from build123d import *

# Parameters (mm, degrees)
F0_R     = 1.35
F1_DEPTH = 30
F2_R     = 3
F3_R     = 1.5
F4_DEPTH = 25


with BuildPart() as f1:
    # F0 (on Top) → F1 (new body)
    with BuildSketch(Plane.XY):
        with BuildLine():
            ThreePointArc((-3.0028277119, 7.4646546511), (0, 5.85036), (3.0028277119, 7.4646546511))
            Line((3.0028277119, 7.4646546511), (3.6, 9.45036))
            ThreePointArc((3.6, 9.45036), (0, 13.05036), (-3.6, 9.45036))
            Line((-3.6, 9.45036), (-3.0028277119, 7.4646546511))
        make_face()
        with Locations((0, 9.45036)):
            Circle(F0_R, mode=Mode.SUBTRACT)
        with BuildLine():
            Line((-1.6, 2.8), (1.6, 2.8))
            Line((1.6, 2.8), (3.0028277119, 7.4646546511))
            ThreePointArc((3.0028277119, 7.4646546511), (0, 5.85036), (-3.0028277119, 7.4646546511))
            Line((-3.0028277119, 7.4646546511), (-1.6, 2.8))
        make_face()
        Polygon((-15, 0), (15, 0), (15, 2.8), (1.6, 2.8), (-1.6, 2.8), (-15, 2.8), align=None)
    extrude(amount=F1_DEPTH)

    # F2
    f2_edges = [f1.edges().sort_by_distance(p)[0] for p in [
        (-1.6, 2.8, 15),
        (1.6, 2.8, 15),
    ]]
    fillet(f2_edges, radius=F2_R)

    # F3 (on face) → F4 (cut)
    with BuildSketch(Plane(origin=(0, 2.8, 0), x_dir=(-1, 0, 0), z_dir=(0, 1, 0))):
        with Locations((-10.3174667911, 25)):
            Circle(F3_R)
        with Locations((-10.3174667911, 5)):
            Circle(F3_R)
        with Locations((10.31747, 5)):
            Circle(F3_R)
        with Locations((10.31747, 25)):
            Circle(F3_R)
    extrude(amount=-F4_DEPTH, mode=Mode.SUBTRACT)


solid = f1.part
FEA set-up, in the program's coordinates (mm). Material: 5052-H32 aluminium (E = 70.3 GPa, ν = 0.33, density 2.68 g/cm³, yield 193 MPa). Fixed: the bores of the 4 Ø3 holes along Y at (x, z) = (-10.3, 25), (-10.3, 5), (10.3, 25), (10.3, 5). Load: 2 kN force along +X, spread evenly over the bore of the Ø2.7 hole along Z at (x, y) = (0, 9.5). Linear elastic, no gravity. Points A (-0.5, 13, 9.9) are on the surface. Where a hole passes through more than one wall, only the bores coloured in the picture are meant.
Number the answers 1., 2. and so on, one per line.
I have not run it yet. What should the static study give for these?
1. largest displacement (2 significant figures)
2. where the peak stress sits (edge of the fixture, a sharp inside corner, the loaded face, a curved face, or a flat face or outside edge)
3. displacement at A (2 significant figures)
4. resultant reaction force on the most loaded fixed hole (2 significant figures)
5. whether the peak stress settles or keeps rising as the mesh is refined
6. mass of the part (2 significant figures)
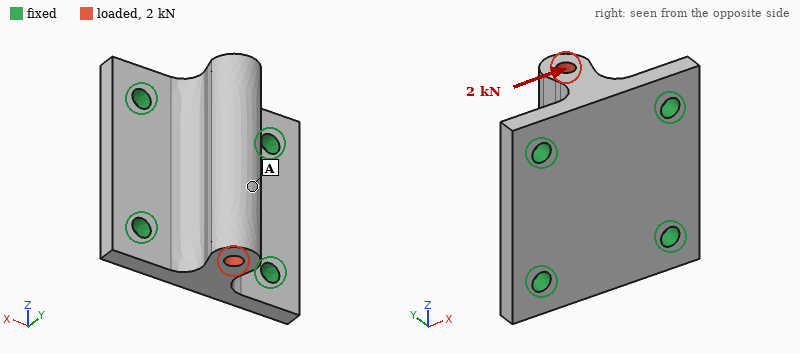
1. 39 µm
2. edge of the fixture
3. 38 µm
4. 720 N
5. keeps rising
6. 11 g
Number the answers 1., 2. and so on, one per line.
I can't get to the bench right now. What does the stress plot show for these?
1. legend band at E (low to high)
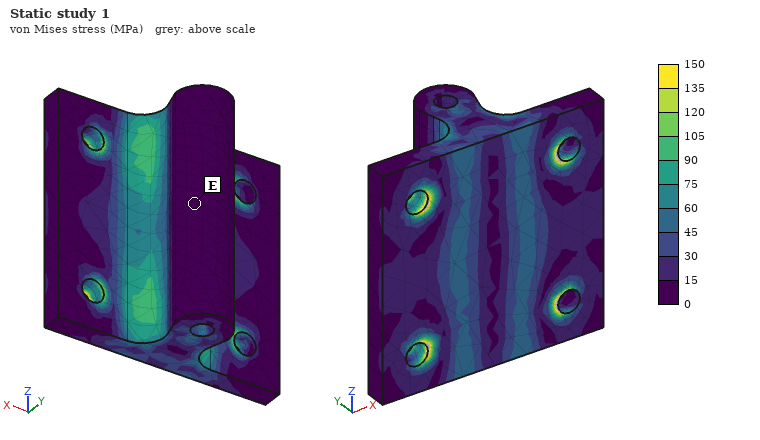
1. 0 to 15 MPa
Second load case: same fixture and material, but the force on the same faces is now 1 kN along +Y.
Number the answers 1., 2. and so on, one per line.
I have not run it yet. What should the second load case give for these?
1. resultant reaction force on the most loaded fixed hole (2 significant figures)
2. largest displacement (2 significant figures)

1. 270 N
2. 8.4 µm
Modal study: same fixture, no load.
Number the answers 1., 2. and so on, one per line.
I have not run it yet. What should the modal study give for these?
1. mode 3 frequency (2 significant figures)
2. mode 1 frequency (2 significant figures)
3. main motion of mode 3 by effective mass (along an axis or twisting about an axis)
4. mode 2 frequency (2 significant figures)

1. 23 kHz
2. 21 kHz
3. along X
4. 21 kHz
